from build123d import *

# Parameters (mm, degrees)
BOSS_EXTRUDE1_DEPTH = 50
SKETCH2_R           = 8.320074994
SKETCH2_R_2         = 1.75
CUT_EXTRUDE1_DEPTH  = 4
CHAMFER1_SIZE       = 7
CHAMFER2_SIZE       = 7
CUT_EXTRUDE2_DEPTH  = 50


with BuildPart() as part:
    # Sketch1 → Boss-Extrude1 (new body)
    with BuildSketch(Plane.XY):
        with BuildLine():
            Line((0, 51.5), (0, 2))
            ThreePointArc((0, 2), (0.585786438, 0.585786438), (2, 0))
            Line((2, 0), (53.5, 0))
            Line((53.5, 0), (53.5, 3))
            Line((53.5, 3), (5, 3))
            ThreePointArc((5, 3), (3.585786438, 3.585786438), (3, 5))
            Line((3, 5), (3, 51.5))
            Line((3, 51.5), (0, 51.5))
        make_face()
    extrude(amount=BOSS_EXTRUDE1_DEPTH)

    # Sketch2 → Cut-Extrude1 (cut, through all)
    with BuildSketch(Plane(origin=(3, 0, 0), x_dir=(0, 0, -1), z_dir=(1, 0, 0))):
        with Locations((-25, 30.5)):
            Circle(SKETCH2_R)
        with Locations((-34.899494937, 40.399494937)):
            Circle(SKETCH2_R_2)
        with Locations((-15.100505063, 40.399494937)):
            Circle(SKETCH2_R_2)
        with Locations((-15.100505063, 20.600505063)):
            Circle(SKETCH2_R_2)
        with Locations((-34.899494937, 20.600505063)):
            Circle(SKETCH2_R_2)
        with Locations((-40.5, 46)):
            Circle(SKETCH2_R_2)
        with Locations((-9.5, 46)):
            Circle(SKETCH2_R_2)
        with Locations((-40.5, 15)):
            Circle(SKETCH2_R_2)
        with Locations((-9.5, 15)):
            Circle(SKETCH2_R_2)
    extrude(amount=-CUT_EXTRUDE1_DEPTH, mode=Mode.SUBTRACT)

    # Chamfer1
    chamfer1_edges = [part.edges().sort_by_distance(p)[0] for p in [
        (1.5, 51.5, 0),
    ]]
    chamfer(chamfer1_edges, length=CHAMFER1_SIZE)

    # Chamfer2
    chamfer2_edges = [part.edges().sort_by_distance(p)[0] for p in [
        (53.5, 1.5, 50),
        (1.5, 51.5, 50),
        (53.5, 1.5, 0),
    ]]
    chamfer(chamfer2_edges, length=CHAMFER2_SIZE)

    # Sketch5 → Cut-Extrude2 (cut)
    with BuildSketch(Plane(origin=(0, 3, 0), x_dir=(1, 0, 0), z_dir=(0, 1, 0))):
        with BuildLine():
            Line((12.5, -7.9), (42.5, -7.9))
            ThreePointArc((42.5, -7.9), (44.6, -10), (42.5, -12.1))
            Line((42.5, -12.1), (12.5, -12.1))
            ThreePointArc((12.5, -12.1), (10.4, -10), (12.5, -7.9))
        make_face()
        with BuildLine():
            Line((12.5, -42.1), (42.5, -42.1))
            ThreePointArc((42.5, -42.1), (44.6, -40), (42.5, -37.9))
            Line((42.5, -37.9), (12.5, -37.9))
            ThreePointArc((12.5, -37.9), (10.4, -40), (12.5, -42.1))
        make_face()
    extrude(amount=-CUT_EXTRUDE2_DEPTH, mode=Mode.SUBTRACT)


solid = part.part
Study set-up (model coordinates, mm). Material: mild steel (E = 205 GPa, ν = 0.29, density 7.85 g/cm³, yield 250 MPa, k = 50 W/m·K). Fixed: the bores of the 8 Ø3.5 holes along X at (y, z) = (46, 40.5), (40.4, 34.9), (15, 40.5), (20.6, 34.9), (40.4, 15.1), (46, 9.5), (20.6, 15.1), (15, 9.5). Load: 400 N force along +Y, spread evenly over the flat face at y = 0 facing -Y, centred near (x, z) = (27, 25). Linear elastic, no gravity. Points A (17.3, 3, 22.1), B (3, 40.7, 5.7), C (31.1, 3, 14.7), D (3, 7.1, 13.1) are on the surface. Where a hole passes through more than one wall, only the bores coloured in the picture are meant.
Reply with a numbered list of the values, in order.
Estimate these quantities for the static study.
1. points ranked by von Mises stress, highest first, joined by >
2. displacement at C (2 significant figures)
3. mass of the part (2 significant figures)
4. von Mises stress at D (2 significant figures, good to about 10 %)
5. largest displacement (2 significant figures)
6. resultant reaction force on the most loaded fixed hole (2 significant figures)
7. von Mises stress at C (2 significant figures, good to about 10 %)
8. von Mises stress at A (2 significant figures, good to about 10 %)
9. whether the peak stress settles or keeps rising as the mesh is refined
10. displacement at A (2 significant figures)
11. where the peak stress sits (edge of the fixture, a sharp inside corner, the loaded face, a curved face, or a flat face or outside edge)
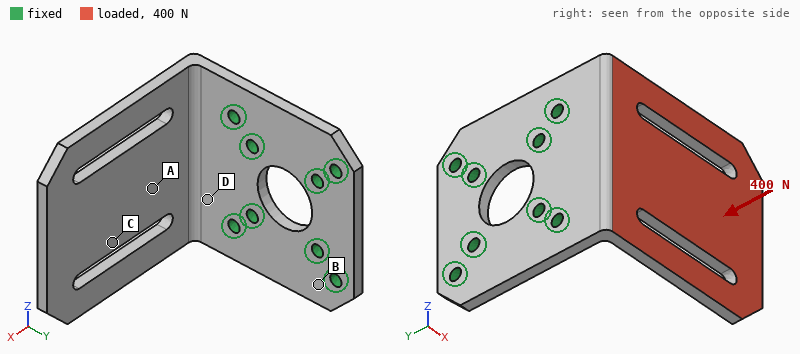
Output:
1. D > A > C > B
2. 0.28 mm
3. 100 g
4. 130 MPa
5. 0.57 mm
6. 260 N
7. 32 MPa
8. 75 MPa
9. keeps rising
10. 0.12 mm
11. edge of the fixture
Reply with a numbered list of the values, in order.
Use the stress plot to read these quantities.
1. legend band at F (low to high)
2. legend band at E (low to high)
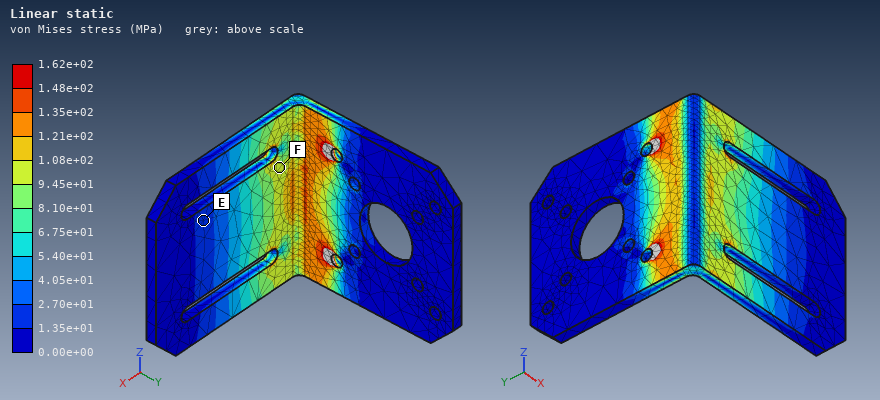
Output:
1. 9.45e+01 to 1.08e+02 MPa
2. 1.35e+01 to 2.70e+01 MPa
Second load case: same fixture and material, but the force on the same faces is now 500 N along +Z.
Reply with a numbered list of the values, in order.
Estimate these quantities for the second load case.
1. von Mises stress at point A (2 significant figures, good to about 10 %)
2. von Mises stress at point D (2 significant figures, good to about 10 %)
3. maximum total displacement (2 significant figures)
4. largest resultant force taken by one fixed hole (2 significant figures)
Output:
1. 12 MPa
2. 49 MPa
3. 62 µm
4. 510 N
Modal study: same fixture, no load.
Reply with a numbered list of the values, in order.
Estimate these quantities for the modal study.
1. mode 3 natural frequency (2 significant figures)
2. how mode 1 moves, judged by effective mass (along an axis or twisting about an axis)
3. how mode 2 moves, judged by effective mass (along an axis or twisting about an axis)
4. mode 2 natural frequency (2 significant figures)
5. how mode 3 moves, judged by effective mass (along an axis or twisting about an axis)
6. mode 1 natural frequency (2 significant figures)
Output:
1. 2700 Hz
2. along Y
3. along Z
4. 1900 Hz
5. along Z
6. 710 Hz
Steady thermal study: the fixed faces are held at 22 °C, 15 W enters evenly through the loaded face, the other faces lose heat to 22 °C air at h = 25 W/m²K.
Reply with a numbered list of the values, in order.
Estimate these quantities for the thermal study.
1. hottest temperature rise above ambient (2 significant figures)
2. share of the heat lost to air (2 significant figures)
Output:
1. 62 K
2. 28 %
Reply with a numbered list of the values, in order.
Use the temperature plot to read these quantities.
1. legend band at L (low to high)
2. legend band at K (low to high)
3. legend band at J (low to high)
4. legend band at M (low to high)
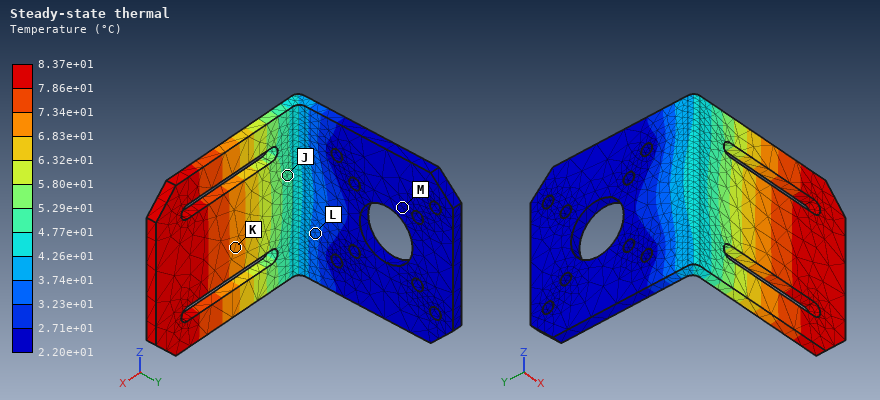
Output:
1. 3.23e+01 to 3.74e+01 °C
2. 6.83e+01 to 7.34e+01 °C
3. 4.77e+01 to 5.29e+01 °C
4. 2.20e+01 to 2.71e+01 °C
